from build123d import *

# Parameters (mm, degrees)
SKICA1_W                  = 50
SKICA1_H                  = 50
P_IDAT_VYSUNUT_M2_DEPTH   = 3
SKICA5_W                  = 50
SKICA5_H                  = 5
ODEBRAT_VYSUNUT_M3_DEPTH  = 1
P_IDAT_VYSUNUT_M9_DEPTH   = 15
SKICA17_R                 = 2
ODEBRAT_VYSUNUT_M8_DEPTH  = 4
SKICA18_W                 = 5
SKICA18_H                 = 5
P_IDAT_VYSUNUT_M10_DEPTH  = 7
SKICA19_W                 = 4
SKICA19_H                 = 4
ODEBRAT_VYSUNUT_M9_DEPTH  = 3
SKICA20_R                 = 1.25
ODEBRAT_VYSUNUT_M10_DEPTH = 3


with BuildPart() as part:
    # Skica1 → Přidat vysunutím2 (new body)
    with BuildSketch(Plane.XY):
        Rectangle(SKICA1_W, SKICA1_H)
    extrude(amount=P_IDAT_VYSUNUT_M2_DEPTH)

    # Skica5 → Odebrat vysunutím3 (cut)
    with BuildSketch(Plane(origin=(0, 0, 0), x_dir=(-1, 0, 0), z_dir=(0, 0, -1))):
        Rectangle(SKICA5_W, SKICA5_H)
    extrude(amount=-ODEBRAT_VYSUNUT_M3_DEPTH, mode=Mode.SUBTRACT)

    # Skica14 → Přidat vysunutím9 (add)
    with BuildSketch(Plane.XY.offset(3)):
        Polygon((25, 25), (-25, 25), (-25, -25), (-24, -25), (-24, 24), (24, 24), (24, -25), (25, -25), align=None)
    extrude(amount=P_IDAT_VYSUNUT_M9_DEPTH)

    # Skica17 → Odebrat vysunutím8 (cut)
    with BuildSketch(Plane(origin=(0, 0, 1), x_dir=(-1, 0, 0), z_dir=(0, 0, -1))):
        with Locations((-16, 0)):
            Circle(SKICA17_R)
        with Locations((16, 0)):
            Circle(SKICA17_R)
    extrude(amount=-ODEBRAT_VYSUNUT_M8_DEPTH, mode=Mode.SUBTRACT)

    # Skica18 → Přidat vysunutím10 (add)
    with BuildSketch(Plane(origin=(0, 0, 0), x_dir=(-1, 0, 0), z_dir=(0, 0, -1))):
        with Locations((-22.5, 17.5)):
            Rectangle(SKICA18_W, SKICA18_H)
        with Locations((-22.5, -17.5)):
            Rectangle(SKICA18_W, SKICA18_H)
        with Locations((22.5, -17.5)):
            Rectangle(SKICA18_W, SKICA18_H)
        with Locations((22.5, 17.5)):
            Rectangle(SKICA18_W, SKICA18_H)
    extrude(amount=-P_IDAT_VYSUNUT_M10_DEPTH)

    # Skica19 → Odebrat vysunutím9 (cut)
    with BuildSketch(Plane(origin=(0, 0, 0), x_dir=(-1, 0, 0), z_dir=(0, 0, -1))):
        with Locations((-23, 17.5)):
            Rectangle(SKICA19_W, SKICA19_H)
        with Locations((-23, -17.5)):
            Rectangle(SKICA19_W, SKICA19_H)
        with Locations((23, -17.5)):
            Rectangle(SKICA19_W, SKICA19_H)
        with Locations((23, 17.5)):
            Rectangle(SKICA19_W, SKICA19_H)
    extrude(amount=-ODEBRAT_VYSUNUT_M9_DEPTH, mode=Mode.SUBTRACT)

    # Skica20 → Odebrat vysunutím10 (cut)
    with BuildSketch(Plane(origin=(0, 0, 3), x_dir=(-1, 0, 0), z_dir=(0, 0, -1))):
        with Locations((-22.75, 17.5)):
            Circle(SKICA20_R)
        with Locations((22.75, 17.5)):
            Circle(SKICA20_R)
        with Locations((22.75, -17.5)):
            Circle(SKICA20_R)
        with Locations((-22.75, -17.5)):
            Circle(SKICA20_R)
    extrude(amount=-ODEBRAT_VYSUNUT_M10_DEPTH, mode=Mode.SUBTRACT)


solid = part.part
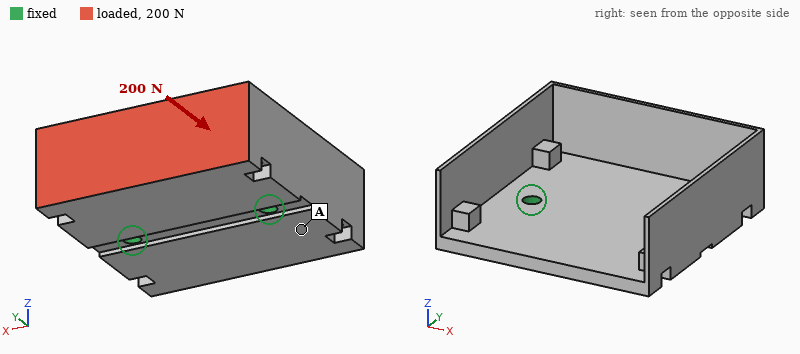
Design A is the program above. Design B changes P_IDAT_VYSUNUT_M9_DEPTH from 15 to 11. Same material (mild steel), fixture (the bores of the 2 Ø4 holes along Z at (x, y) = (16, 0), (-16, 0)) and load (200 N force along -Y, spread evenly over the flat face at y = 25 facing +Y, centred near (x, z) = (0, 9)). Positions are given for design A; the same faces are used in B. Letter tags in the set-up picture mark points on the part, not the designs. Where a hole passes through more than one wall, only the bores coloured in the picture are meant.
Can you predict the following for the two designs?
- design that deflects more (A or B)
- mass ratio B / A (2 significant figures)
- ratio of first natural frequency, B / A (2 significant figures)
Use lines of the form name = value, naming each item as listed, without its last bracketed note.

design that deflects more = A
mass ratio B / A = 0.94
ratio of first natural frequency, B / A = 1.1
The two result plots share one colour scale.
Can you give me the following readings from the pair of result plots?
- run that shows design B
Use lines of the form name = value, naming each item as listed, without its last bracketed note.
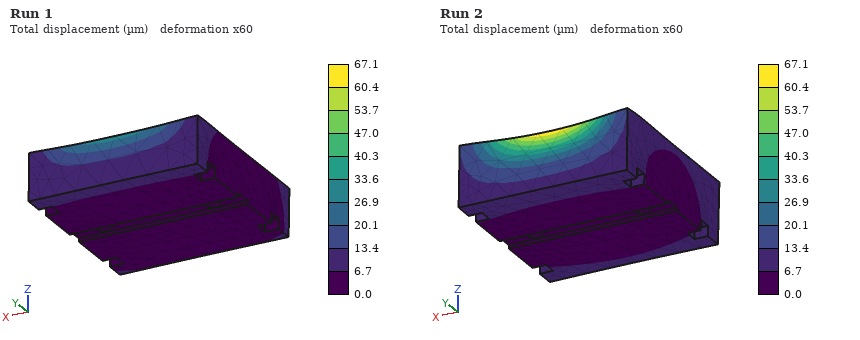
run that shows design B = Run 1
